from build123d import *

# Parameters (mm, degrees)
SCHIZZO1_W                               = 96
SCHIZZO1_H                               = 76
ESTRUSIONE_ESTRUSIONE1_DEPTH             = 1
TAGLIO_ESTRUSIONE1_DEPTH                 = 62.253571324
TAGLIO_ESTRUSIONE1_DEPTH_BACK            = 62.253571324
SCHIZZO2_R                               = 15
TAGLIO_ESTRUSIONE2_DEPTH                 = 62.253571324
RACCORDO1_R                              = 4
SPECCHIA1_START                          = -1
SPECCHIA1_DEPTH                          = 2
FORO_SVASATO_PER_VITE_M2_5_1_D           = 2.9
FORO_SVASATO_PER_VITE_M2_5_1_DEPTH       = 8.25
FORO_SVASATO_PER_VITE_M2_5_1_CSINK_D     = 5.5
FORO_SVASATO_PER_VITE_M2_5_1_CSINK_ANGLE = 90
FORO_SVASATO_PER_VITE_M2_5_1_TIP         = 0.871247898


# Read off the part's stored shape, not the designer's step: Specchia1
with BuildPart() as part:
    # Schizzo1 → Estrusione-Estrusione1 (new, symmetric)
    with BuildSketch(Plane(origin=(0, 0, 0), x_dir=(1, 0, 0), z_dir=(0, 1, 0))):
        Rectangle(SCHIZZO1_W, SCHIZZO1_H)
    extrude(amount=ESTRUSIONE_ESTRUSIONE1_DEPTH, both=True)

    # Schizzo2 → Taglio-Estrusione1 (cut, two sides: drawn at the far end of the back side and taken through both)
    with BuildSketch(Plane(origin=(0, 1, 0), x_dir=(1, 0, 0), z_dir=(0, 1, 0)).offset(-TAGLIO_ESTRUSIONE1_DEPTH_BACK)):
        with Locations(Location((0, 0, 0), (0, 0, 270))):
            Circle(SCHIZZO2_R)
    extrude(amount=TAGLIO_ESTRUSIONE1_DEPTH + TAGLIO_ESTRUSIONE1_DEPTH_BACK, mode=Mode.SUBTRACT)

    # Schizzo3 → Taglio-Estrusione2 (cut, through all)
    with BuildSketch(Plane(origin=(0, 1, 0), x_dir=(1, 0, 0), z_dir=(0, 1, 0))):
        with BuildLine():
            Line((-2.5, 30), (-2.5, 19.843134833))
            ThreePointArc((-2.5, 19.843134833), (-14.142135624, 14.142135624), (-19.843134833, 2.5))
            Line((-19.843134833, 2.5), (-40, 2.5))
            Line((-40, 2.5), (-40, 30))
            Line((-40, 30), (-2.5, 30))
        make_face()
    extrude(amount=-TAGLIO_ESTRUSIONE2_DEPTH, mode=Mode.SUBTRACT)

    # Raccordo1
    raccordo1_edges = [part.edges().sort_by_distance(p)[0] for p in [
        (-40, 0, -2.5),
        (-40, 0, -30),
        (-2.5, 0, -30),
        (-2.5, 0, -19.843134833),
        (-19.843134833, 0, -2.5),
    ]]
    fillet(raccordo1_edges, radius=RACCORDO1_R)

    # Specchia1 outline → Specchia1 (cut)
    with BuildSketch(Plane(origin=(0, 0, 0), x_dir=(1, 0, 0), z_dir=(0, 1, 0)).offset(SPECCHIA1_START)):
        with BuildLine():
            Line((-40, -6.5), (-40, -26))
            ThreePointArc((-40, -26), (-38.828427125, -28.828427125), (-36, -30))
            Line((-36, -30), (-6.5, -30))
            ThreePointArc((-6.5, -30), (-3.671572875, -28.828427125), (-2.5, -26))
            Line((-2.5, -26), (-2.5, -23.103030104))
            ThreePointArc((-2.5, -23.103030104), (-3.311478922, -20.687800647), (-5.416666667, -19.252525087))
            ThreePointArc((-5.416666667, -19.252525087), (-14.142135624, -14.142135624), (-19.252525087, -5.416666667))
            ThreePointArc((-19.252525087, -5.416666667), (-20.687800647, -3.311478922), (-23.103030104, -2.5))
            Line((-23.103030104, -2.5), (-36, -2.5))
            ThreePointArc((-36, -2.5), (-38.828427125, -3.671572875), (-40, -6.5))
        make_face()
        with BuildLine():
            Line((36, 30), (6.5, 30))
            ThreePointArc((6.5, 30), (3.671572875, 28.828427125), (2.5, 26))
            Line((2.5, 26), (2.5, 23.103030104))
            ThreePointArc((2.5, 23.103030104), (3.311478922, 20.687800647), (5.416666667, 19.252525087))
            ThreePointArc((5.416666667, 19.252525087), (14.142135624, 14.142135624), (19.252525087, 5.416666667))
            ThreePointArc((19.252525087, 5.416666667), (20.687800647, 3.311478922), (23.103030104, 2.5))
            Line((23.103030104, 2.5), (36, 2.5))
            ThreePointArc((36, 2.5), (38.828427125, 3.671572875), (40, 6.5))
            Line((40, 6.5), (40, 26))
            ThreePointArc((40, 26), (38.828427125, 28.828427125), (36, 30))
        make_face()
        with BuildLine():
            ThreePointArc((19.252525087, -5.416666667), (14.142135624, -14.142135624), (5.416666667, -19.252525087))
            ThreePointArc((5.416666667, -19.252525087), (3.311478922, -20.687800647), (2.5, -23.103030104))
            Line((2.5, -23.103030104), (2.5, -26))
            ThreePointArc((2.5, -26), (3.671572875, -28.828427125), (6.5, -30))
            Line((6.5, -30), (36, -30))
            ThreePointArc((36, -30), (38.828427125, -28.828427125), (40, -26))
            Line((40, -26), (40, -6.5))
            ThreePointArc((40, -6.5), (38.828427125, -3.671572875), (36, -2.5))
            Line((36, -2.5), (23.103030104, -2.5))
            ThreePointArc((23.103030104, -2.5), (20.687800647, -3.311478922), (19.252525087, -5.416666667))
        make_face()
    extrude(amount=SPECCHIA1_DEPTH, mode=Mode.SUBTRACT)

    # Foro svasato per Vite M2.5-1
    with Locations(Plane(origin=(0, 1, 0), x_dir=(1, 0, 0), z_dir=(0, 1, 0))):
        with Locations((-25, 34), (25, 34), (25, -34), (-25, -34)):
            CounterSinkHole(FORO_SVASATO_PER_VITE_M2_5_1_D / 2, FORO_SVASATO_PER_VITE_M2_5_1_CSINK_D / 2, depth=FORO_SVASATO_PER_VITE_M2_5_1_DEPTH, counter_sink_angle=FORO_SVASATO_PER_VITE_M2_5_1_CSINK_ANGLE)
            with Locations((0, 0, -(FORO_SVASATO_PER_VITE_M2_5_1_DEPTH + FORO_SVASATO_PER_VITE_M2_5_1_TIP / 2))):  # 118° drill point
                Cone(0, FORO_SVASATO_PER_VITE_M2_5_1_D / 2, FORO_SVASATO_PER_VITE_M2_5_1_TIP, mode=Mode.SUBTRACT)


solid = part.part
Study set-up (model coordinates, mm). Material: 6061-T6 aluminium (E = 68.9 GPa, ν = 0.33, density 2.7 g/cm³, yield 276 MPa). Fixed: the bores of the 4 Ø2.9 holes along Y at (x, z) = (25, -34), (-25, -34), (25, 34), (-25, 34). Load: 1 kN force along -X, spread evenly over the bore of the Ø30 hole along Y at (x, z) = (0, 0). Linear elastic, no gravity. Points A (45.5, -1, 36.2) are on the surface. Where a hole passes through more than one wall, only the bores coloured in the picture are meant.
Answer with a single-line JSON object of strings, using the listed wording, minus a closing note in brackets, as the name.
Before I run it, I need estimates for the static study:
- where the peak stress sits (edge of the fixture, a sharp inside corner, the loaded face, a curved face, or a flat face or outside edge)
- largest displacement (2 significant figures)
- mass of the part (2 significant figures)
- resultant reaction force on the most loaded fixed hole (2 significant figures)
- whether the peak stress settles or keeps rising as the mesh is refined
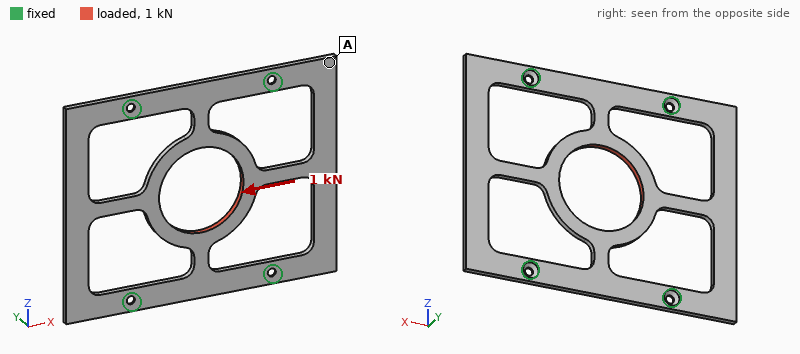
{"where the peak stress sits": "edge of the fixture", "largest displacement": "73 µm", "mass of the part": "18 g", "resultant reaction force on the most loaded fixed hole": "250 N", "whether the peak stress settles or keeps rising as the mesh is refined": "keeps rising"}
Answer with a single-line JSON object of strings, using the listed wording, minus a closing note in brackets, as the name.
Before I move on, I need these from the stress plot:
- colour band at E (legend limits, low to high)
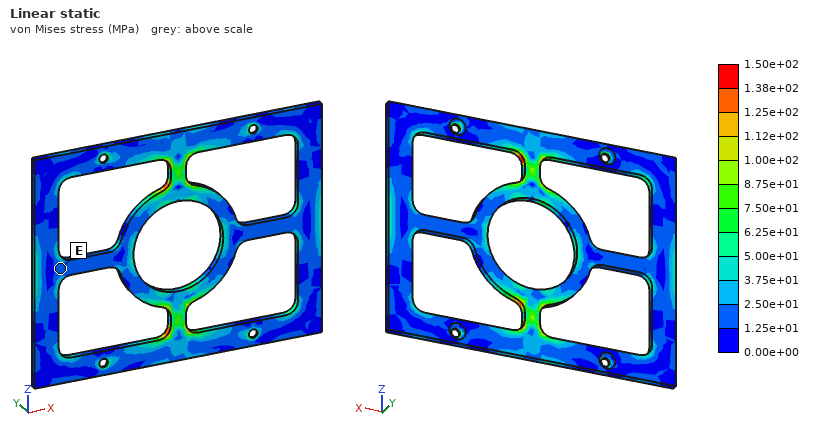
{"colour band at E": "1.25e+01 to 2.50e+01 MPa"}
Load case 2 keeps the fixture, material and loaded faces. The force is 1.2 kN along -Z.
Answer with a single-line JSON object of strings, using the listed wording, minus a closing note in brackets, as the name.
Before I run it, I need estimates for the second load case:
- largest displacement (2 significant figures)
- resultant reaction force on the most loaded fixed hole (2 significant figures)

{"largest displacement": "0.12 mm", "resultant reaction force on the most loaded fixed hole": "310 N"}
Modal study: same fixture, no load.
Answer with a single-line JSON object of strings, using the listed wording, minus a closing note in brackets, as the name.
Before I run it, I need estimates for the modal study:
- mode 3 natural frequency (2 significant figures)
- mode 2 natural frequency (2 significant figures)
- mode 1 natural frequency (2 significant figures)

{"mode 3 natural frequency": "1500 Hz", "mode 2 natural frequency": "1100 Hz", "mode 1 natural frequency": "1000 Hz"}
